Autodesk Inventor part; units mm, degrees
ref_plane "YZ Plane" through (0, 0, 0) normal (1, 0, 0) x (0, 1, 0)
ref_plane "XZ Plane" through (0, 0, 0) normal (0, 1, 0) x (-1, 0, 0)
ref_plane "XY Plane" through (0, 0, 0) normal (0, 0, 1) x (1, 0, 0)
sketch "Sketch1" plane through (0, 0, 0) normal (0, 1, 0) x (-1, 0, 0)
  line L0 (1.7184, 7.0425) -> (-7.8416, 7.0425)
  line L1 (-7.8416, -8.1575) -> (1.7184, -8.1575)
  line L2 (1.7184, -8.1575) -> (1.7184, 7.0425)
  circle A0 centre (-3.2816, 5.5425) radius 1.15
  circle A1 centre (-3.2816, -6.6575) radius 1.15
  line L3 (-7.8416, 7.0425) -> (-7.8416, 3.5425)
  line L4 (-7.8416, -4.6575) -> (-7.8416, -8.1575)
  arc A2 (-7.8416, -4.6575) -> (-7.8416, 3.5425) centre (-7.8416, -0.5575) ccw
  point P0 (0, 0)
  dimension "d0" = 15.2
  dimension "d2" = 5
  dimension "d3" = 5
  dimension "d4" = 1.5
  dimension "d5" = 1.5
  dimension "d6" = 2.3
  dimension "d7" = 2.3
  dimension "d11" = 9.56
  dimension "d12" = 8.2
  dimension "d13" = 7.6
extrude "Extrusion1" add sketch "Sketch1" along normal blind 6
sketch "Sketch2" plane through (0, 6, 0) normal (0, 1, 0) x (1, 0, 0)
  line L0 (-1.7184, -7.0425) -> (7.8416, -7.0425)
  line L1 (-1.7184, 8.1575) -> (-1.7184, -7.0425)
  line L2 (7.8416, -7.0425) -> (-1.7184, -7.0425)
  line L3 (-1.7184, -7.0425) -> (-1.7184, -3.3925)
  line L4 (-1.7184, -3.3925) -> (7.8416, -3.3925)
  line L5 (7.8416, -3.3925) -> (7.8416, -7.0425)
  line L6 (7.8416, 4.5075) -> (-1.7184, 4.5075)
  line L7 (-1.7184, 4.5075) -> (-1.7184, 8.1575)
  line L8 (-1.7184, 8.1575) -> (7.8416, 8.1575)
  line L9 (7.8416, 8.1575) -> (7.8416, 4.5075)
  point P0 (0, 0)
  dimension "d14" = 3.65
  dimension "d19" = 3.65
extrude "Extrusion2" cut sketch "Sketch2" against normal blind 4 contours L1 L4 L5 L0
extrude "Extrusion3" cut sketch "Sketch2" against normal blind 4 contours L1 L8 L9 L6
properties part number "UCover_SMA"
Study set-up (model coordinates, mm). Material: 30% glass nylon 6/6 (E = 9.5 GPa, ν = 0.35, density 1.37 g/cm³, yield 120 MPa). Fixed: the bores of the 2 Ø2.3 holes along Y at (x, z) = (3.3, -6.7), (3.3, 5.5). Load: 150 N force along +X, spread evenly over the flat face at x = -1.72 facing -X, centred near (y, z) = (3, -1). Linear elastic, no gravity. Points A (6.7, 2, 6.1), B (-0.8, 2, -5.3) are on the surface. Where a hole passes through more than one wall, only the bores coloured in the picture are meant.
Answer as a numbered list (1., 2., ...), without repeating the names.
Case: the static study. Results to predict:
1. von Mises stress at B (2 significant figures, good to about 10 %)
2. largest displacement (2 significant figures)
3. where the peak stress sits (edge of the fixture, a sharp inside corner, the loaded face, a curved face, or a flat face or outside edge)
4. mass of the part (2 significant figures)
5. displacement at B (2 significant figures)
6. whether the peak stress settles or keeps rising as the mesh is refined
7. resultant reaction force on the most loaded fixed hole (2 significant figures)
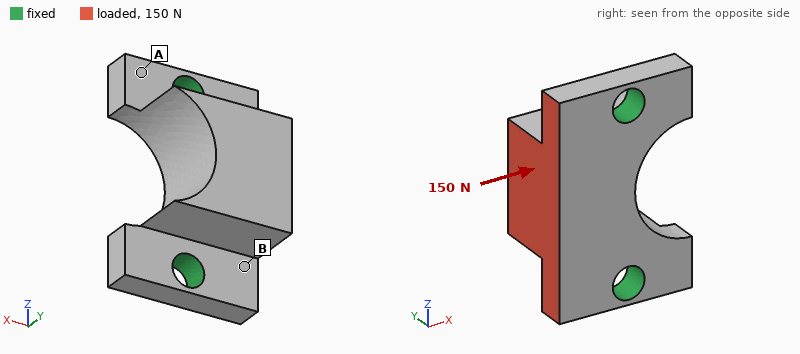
1. 8.9 MPa
2. 30 µm
3. edge of the fixture
4. 0.57 g
5. 12 µm
6. keeps rising
7. 81 N
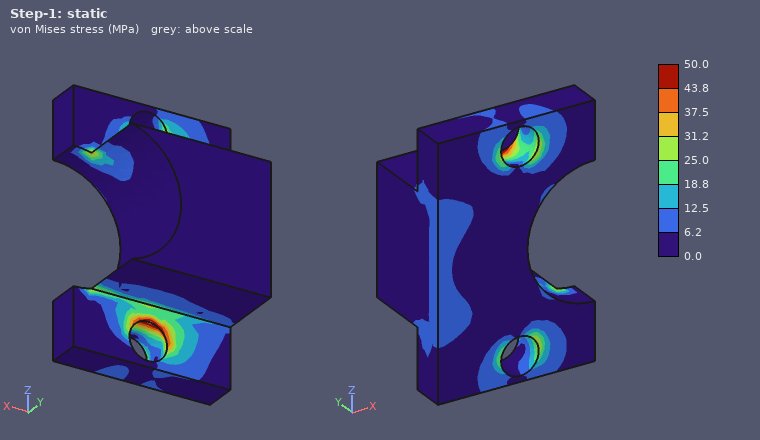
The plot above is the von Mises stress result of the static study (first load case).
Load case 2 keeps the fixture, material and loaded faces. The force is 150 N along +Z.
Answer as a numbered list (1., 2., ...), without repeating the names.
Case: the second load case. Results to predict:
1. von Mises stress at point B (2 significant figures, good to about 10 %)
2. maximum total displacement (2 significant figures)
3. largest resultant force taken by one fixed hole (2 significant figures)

1. 10 MPa
2. 12 µm
3. 97 N
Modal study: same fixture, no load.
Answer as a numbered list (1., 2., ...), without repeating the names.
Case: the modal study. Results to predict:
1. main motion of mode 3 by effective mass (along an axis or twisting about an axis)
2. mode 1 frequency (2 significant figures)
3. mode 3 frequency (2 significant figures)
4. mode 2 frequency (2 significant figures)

1. along Z
2. 16 kHz
3. 37 kHz
4. 34 kHz
